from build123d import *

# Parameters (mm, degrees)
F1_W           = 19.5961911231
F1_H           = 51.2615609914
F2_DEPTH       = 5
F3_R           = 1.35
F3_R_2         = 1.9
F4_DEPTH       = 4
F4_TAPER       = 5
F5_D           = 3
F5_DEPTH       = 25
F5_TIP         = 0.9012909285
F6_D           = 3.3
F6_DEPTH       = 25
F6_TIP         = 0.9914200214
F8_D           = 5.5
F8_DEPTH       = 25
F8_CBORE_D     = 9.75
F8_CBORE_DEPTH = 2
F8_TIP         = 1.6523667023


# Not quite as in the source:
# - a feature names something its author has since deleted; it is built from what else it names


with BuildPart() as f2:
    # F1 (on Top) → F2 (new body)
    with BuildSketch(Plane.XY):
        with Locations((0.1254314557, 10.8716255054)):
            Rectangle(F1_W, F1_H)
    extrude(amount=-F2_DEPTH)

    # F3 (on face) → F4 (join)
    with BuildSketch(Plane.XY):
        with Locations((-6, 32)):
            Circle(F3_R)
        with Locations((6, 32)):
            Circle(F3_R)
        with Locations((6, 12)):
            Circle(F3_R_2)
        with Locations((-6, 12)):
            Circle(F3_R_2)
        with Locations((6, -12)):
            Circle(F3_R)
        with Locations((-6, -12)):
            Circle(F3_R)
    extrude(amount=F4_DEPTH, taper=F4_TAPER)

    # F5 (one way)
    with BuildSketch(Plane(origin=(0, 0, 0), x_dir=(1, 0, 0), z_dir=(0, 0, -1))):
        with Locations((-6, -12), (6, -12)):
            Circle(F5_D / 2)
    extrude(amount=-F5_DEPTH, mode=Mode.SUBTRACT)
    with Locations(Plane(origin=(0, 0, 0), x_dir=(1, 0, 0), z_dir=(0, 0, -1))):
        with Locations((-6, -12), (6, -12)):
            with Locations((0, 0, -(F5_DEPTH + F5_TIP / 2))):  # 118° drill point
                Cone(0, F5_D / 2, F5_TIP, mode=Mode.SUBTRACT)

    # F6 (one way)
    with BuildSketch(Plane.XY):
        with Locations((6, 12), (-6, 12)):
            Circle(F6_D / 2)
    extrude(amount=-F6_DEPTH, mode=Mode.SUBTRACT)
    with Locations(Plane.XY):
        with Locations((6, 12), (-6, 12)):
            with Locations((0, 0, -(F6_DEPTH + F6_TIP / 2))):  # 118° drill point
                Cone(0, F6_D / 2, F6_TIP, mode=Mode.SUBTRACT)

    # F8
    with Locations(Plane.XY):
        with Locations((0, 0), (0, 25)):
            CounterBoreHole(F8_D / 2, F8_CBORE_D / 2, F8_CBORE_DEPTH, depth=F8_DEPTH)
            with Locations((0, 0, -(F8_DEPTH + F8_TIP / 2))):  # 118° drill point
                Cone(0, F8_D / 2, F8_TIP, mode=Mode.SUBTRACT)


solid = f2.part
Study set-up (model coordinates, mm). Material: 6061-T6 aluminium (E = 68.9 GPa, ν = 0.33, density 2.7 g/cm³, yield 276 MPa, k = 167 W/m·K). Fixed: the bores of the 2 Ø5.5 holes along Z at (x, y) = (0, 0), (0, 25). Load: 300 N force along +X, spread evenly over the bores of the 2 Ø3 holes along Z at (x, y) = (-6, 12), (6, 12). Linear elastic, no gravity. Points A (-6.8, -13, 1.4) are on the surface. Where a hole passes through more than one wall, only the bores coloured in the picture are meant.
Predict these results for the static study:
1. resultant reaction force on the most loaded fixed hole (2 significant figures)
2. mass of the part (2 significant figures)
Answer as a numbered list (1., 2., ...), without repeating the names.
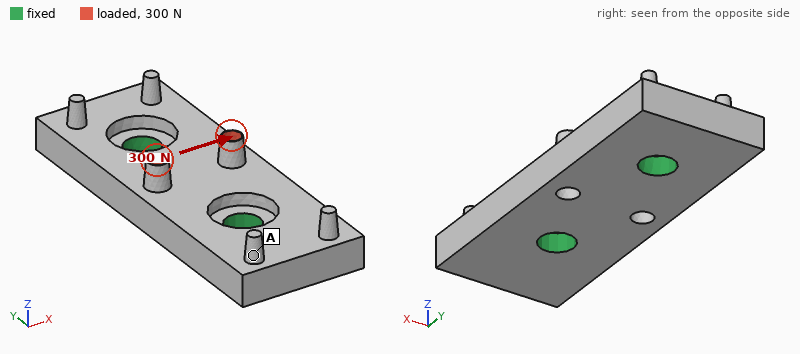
1. 160 N
2. 12 g
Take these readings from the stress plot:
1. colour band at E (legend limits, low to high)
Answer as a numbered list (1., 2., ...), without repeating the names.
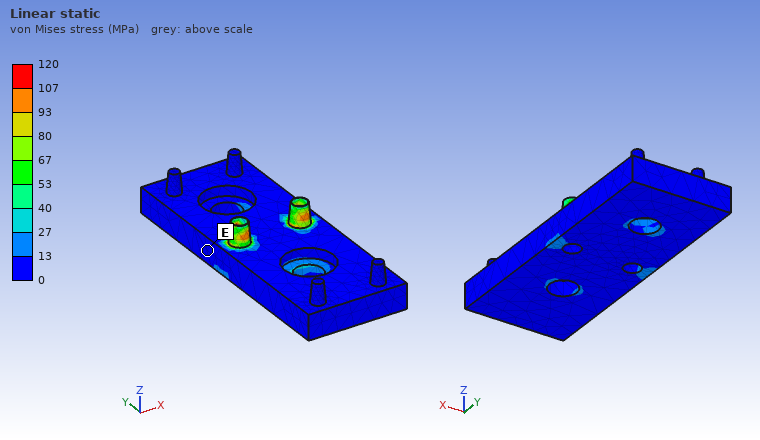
1. 0 to 13 MPa
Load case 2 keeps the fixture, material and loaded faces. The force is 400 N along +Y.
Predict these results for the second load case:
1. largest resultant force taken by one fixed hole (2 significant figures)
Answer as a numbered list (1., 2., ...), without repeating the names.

1. 230 N
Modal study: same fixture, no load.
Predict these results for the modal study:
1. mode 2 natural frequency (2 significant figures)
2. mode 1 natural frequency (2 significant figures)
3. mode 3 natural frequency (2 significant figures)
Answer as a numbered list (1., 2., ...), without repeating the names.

1. 18 kHz
2. 14 kHz
3. 21 kHz
